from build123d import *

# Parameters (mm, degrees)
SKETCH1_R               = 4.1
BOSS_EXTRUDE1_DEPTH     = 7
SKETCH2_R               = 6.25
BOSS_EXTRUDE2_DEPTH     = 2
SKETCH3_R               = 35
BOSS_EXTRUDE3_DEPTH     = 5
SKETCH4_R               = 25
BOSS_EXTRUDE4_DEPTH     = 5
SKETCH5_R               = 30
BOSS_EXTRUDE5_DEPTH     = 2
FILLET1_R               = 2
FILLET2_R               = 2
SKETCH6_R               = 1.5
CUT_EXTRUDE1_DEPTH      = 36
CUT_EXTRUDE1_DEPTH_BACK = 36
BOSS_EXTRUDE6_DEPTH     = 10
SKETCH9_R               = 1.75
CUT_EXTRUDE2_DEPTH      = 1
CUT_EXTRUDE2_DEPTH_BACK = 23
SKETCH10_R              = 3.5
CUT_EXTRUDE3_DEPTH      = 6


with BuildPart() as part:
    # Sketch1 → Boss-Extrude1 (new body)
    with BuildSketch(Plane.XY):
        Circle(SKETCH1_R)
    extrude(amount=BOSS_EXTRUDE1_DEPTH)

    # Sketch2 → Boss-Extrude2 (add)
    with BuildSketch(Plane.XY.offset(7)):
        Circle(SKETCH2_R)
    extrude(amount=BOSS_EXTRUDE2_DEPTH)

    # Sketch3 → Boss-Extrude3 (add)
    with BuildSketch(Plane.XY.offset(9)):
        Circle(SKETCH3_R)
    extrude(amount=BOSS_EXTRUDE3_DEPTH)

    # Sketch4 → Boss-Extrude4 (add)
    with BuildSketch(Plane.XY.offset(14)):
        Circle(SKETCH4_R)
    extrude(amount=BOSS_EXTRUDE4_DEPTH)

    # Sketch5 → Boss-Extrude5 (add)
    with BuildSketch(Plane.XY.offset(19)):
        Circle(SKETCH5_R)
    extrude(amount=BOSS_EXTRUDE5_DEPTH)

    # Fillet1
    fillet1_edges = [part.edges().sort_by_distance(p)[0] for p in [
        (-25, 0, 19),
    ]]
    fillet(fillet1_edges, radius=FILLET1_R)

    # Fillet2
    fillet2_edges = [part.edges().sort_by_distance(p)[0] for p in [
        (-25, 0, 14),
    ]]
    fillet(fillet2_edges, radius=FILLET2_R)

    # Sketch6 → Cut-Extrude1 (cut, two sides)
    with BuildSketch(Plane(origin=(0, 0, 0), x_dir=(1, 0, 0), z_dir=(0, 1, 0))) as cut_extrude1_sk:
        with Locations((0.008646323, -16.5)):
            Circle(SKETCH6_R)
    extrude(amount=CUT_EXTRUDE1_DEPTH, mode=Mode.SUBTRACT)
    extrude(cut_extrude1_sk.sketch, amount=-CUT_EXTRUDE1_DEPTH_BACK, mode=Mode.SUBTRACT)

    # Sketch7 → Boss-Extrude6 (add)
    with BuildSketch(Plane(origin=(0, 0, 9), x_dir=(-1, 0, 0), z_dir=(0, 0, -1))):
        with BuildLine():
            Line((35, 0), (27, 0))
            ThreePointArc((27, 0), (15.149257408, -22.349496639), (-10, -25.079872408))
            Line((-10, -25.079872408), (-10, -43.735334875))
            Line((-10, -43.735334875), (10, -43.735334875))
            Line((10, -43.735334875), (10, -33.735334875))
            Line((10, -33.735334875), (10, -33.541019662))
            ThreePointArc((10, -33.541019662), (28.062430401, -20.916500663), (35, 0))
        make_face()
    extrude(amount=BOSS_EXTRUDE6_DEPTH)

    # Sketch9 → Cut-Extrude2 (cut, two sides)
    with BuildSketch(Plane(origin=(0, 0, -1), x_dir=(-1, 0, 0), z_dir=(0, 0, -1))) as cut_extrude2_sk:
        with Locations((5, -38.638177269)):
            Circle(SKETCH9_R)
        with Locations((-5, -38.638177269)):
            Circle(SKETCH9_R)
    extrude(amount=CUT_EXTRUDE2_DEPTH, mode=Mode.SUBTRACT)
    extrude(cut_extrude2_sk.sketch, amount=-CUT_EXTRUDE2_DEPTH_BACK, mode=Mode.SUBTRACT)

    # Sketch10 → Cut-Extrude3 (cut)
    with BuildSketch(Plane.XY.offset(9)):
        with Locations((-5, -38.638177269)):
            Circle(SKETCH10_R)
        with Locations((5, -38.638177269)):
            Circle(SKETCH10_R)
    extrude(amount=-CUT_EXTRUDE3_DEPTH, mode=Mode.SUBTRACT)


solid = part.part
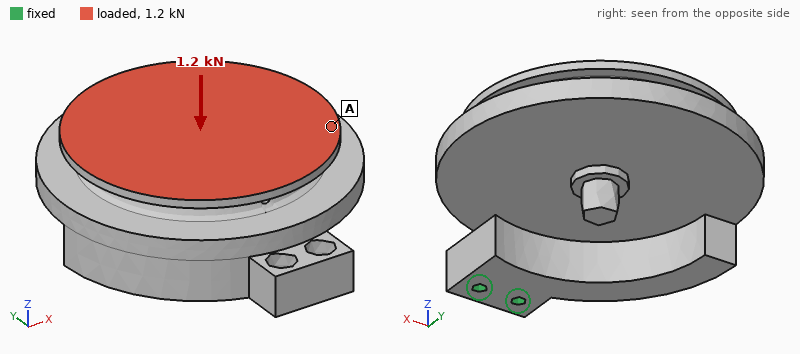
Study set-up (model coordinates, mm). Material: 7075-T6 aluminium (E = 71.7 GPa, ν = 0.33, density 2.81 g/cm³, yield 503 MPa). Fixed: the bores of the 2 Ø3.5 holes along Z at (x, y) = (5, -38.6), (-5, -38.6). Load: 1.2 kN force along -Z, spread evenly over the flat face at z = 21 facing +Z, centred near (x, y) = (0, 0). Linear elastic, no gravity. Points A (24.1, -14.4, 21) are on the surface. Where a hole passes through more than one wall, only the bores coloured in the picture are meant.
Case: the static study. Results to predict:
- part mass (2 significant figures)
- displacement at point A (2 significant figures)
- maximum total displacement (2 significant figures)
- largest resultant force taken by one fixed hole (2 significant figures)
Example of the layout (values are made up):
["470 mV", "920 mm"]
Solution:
["120 g", "0.39 mm", "1.1 mm", "610 N"]
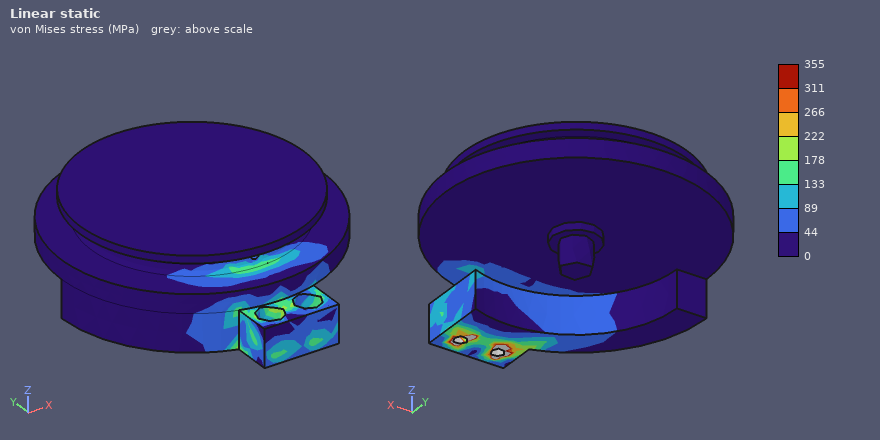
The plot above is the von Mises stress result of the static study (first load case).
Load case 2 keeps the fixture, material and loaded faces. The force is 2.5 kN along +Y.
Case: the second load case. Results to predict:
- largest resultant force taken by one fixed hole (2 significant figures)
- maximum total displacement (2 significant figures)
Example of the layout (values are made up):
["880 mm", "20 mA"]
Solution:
["1.3 kN", "1.1 mm"]
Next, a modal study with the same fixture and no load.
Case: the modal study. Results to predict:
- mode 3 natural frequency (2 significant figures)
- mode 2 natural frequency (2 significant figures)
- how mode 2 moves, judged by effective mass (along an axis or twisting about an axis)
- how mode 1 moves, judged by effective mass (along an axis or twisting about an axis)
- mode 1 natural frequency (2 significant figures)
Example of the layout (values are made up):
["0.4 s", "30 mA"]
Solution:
["2300 Hz", "1300 Hz", "along X", "along Z", "660 Hz"]
